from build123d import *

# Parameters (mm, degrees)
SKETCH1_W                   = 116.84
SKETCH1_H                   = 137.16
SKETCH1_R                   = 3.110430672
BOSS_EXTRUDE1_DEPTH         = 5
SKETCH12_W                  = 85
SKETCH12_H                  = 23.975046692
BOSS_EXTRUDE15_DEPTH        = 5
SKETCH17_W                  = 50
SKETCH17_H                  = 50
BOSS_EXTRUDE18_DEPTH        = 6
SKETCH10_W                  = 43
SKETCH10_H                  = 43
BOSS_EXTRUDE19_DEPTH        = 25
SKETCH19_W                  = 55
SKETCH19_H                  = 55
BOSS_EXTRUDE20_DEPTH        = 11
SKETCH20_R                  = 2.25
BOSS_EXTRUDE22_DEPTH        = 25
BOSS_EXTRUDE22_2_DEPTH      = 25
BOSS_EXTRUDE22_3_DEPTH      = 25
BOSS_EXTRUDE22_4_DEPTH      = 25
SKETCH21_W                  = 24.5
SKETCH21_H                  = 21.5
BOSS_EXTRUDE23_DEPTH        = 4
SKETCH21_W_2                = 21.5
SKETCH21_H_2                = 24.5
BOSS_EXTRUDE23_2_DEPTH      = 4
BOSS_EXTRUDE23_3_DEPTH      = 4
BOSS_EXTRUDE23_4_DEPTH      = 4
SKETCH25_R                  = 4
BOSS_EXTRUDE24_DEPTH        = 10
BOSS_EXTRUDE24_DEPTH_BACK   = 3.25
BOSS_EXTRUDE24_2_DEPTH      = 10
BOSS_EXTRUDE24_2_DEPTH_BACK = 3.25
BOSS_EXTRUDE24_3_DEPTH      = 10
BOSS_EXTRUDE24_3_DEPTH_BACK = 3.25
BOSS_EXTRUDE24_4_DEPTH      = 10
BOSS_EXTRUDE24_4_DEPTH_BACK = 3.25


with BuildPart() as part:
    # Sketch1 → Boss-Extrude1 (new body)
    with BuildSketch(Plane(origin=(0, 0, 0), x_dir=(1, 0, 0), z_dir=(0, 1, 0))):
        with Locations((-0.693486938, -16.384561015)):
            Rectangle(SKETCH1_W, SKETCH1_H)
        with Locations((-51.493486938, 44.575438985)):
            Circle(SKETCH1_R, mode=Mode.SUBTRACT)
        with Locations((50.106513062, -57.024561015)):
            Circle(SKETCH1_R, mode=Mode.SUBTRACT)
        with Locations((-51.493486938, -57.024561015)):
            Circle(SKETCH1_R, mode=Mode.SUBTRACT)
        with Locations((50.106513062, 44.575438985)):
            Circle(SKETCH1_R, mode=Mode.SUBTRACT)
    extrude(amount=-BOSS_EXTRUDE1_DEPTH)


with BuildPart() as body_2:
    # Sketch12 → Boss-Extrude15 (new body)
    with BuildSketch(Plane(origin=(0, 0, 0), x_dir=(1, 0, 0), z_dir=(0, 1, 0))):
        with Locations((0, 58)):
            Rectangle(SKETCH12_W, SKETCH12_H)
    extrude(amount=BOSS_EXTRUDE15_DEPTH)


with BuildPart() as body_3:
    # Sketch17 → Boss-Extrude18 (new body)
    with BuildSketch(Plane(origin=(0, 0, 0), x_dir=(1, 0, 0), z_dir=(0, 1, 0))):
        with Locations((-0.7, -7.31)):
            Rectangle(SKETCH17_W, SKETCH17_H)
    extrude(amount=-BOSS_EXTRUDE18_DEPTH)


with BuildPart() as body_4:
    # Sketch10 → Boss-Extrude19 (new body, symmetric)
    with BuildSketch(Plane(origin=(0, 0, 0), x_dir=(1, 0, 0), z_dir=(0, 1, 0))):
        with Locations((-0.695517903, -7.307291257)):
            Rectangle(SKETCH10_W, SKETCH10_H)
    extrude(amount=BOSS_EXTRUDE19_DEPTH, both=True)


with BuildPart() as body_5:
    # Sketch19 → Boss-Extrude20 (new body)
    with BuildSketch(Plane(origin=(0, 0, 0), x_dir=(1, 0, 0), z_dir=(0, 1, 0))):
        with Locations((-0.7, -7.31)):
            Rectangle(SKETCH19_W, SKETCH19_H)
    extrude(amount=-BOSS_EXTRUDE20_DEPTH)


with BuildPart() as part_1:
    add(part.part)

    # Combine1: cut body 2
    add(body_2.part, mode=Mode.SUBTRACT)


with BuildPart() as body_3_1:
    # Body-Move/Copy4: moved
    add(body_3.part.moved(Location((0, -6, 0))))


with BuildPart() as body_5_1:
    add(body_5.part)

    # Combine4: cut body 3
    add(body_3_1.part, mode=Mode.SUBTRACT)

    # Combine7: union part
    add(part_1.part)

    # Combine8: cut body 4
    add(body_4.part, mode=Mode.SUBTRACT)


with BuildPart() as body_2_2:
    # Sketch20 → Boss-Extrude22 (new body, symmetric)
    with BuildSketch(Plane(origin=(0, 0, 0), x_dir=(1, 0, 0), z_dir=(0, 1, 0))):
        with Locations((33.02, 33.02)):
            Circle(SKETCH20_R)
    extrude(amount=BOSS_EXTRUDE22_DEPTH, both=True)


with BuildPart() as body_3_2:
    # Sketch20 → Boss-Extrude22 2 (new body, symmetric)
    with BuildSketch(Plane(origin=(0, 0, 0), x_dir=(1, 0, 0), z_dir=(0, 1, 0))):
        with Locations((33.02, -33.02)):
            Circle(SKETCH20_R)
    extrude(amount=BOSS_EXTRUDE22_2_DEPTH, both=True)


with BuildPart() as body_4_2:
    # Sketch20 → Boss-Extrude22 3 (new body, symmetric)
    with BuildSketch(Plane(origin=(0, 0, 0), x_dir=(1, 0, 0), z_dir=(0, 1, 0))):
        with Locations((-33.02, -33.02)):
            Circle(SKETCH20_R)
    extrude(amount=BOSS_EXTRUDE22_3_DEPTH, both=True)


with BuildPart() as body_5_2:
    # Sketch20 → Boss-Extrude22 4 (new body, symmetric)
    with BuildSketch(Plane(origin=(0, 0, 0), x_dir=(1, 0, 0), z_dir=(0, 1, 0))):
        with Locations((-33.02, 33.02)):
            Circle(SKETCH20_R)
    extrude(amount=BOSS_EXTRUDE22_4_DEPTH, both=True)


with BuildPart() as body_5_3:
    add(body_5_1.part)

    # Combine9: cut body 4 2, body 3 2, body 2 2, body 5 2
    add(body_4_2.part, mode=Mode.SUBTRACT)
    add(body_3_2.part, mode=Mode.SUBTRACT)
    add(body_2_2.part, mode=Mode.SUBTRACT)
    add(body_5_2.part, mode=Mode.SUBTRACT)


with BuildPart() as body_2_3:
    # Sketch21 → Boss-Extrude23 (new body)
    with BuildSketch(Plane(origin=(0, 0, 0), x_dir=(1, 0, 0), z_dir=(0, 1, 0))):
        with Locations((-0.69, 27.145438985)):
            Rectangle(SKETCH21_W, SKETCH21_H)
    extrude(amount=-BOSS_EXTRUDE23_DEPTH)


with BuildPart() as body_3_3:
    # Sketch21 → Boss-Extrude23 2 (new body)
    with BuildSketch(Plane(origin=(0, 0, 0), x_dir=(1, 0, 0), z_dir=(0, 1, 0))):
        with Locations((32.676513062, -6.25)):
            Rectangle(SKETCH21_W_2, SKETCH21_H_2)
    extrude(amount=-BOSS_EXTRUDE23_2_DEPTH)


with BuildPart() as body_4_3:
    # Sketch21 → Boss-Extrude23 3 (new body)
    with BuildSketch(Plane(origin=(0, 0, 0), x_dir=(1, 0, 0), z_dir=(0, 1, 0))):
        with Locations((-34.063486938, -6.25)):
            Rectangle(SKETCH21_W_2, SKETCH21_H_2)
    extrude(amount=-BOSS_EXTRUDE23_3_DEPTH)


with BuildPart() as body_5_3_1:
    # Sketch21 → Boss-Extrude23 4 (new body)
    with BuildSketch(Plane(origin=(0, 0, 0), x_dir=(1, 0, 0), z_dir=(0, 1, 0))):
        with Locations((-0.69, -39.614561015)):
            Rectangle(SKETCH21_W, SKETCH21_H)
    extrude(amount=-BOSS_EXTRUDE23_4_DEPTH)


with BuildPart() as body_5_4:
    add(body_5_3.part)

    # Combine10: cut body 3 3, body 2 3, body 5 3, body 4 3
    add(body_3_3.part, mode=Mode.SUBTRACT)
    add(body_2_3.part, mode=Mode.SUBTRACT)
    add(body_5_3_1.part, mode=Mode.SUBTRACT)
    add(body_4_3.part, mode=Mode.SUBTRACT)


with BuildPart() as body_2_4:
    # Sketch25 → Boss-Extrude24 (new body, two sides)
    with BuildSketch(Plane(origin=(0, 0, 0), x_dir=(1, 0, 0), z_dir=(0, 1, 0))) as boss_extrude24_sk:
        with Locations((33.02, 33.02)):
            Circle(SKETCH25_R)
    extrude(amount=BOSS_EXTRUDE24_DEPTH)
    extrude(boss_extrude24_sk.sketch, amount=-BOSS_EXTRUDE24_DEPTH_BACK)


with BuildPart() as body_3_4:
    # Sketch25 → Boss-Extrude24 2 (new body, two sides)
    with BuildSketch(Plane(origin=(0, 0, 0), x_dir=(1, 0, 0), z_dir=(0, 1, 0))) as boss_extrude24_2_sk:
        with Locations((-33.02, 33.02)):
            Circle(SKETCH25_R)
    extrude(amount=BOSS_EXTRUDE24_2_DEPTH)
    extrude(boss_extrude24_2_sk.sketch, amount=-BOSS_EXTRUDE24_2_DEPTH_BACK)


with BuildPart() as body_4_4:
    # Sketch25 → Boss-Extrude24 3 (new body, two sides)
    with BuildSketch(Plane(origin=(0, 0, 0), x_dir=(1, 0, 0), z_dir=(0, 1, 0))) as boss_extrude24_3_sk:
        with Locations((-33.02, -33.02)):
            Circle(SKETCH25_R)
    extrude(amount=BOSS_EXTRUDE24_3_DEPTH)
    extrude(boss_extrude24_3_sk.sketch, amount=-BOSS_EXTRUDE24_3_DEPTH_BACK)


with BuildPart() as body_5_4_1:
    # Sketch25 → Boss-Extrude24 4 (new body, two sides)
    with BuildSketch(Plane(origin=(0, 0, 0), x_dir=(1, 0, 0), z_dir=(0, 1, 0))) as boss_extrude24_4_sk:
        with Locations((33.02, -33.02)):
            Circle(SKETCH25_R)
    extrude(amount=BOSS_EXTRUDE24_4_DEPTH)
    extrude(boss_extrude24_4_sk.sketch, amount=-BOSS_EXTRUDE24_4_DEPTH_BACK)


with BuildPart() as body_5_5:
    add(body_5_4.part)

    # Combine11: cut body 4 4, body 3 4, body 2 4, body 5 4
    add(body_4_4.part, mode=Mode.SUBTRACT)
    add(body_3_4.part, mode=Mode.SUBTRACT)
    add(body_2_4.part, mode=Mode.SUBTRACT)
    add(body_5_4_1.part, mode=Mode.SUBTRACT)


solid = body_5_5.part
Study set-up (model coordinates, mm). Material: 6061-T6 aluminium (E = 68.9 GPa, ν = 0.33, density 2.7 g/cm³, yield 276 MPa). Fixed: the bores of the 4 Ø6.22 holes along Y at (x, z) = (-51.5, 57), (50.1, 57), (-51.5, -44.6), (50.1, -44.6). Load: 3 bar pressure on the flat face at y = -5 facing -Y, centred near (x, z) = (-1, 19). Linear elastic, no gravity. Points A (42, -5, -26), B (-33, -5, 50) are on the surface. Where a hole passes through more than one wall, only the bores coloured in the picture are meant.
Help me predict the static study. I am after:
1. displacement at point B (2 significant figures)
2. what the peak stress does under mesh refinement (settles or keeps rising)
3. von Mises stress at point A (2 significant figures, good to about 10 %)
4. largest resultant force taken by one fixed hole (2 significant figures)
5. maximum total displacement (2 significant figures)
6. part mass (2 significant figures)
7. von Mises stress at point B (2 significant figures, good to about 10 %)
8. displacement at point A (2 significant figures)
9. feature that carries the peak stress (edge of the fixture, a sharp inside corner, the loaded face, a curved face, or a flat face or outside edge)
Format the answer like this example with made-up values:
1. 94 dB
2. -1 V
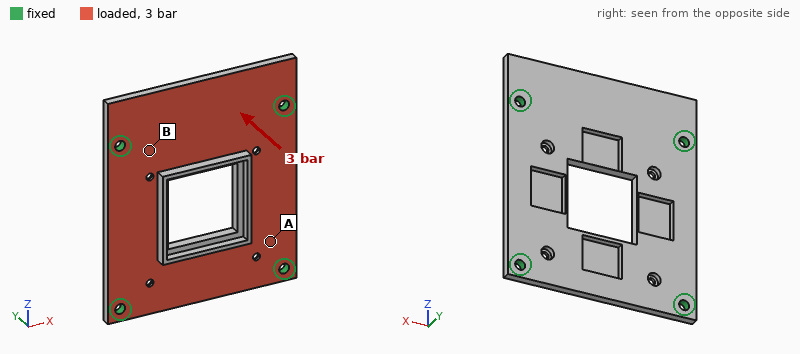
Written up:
1. 0.065 mm
2. keeps rising
3. 14 MPa
4. 1.3 kN
5. 0.17 mm
6. 180 g
7. 28 MPa
8. 0.064 mm
9. edge of the fixture
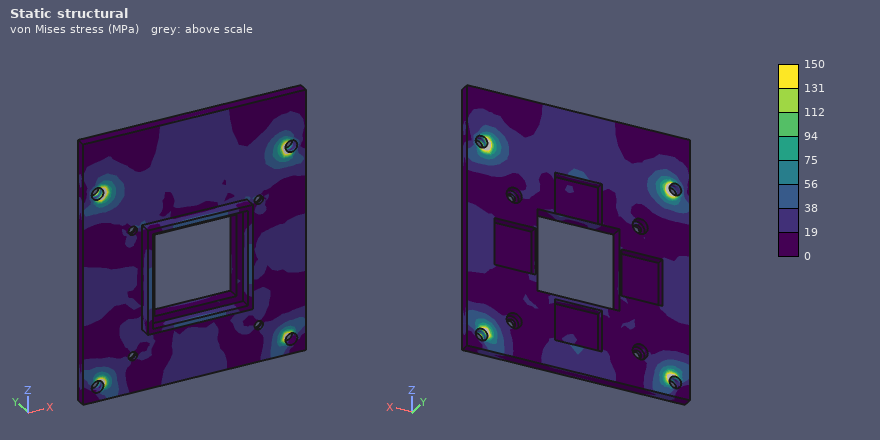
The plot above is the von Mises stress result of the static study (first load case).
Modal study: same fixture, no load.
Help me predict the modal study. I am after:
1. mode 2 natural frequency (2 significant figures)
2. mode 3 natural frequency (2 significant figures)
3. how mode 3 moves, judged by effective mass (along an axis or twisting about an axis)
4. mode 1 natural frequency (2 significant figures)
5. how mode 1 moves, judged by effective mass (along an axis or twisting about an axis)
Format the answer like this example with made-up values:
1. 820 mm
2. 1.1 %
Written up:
1. 2300 Hz
2. 2900 Hz
3. twisting about Z
4. 2100 Hz
5. along Y
